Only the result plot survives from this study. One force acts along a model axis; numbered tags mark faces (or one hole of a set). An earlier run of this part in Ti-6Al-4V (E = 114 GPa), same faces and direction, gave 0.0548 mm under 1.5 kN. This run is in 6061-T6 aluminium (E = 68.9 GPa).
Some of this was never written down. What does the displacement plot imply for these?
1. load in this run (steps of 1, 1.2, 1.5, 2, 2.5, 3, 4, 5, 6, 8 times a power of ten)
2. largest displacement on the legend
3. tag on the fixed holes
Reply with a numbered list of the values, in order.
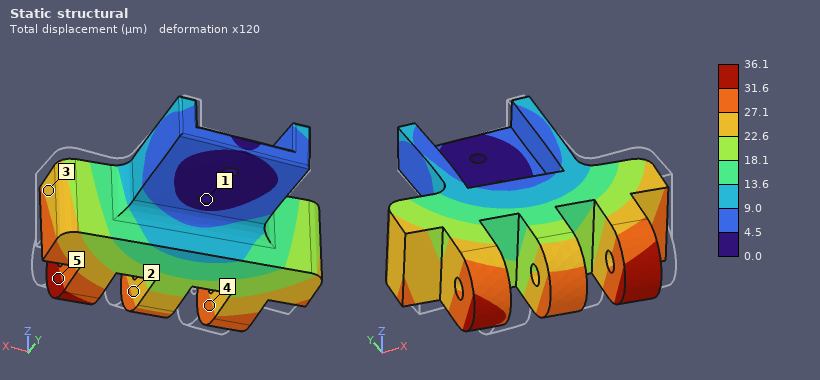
1. 600 N
2. 36.1 µm
3. 1
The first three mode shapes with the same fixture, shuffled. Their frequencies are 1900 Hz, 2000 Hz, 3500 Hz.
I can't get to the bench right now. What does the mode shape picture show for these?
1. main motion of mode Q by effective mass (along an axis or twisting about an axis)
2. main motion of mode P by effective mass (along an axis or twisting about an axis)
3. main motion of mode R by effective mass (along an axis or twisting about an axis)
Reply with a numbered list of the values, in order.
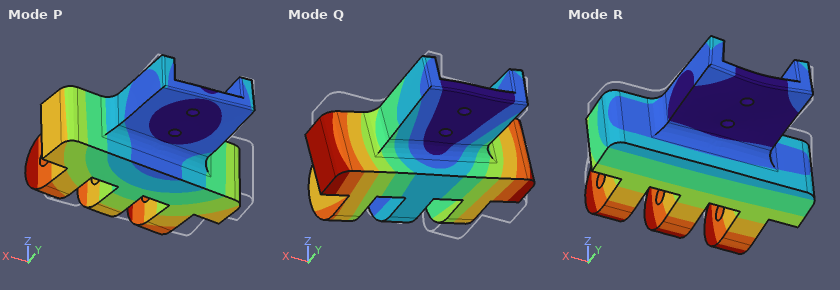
1. twisting about Y
2. along X
3. along Z
